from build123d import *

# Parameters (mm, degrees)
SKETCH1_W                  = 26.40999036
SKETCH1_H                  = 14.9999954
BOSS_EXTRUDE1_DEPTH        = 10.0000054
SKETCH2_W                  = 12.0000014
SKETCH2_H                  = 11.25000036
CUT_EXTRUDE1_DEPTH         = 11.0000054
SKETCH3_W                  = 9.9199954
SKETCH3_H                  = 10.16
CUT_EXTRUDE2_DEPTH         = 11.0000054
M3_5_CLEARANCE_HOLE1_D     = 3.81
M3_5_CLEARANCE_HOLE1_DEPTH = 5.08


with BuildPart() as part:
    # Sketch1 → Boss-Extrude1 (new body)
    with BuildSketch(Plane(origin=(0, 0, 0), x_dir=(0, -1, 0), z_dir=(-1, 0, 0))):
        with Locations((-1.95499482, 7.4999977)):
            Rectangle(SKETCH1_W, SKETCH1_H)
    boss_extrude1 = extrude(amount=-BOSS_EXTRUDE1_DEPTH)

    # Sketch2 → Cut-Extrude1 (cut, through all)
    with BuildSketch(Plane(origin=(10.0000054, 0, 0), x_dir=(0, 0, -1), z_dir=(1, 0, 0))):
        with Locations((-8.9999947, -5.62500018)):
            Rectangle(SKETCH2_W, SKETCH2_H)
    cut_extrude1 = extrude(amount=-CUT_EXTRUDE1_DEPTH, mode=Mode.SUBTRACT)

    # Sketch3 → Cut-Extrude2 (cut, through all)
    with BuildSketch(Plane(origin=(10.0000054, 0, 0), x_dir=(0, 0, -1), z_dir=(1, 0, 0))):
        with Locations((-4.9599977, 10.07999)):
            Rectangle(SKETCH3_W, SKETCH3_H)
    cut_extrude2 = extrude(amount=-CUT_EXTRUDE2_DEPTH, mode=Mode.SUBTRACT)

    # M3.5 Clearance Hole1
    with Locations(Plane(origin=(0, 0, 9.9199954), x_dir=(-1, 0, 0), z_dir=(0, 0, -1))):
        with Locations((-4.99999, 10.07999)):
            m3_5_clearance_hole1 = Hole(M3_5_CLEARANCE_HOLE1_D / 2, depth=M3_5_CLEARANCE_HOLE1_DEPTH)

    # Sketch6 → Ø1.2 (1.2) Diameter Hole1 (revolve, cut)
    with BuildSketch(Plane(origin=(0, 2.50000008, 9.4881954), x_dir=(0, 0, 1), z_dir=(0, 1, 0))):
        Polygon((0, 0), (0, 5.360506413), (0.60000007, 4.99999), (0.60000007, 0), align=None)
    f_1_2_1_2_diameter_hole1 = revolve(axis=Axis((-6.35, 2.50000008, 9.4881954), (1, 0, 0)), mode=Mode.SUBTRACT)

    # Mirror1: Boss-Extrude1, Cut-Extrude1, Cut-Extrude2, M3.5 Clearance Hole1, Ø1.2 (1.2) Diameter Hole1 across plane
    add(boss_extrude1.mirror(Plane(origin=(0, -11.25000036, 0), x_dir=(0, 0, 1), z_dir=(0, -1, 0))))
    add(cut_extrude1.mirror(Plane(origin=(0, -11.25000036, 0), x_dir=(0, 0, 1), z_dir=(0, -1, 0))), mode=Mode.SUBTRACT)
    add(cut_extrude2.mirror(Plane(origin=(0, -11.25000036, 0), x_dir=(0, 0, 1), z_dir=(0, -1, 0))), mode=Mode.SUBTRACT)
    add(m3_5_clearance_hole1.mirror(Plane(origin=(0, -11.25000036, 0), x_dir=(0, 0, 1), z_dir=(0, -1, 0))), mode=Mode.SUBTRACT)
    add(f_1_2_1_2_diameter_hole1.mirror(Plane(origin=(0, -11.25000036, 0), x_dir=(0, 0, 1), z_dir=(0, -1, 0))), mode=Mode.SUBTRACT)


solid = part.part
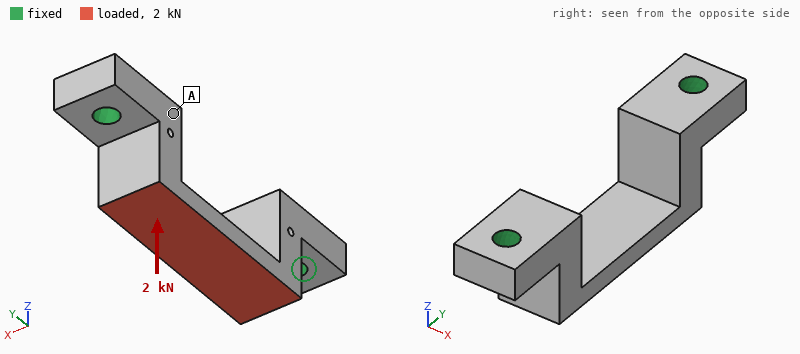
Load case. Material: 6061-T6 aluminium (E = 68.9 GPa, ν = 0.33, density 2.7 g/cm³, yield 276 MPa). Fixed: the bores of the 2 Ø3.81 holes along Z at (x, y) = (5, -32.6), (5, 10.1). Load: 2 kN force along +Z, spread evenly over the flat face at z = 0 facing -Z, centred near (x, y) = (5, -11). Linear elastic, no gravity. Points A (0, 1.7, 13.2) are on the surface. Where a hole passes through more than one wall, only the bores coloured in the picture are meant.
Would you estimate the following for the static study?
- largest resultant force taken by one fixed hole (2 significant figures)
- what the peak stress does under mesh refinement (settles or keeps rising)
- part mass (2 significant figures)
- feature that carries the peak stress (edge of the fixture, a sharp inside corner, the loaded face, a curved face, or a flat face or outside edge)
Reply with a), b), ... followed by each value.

a) 1.2 kN
b) keeps rising
c) 8.3 g
d) edge of the fixture
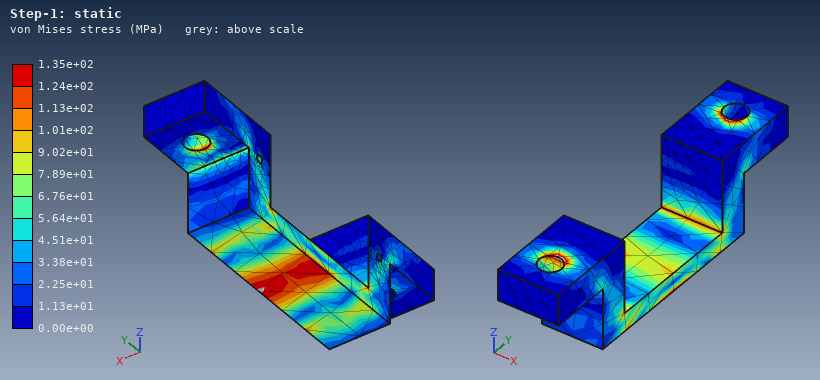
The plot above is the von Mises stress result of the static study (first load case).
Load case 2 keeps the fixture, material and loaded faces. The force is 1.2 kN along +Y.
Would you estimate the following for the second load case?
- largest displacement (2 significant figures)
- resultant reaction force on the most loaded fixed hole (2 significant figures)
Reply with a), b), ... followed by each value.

a) 54 µm
b) 640 N
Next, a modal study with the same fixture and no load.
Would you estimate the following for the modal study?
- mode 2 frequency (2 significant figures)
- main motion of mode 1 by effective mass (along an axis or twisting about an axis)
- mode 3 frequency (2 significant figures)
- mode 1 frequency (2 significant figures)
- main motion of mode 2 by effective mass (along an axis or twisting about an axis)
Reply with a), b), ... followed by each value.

a) 13 kHz
b) along X
c) 18 kHz
d) 11 kHz
e) along Y
